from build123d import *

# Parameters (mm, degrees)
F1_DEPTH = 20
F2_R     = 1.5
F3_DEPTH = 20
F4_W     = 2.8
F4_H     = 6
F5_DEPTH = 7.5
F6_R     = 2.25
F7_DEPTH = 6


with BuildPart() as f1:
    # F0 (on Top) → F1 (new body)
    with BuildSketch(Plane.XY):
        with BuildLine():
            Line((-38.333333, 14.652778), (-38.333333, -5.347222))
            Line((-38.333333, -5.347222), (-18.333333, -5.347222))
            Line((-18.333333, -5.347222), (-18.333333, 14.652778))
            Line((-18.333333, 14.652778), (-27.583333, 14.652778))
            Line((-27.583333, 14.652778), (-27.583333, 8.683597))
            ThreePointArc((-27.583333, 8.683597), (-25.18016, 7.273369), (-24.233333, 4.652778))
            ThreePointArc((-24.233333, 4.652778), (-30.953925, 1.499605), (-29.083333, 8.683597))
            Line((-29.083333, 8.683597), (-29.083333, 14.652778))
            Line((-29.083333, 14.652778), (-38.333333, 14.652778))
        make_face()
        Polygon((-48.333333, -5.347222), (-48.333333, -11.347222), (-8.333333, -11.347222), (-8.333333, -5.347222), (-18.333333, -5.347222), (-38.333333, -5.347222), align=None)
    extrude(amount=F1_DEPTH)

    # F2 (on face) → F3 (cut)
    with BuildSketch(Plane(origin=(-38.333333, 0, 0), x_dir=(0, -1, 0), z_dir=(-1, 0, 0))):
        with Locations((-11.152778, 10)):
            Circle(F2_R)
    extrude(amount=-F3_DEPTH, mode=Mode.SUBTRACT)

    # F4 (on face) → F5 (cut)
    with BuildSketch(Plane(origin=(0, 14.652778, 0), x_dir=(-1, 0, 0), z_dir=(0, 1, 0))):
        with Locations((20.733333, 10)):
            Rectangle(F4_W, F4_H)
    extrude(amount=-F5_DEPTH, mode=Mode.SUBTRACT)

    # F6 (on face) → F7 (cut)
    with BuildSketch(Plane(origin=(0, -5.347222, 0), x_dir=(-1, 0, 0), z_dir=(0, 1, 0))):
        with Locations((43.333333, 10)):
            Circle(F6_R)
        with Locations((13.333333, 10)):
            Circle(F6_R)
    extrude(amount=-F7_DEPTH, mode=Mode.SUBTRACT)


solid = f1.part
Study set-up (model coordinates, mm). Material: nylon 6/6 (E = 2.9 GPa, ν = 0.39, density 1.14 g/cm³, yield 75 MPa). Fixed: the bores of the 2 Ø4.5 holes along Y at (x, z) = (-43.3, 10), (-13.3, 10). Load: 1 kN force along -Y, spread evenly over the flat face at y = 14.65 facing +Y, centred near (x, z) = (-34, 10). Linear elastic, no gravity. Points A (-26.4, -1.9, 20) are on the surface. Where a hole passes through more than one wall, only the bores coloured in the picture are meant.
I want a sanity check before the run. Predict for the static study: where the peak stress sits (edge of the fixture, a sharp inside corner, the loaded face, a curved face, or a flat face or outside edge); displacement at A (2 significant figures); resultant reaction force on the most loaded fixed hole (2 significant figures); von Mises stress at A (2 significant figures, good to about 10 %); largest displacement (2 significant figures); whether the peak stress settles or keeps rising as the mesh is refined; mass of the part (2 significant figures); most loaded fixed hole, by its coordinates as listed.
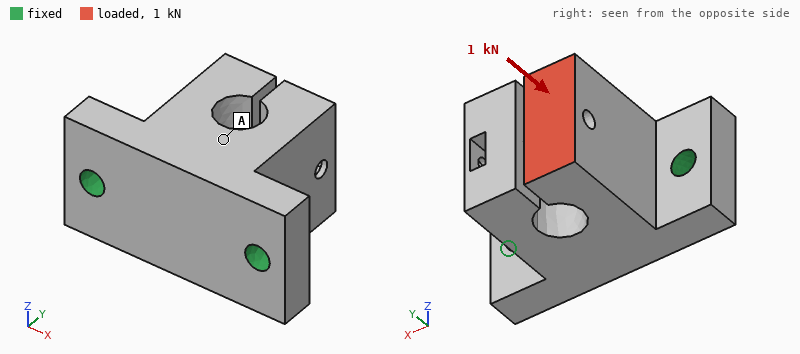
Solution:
edge of the fixture
0.065 mm
740 N
4.9 MPa
0.21 mm
keeps rising
13 g
(-43.3, 10)
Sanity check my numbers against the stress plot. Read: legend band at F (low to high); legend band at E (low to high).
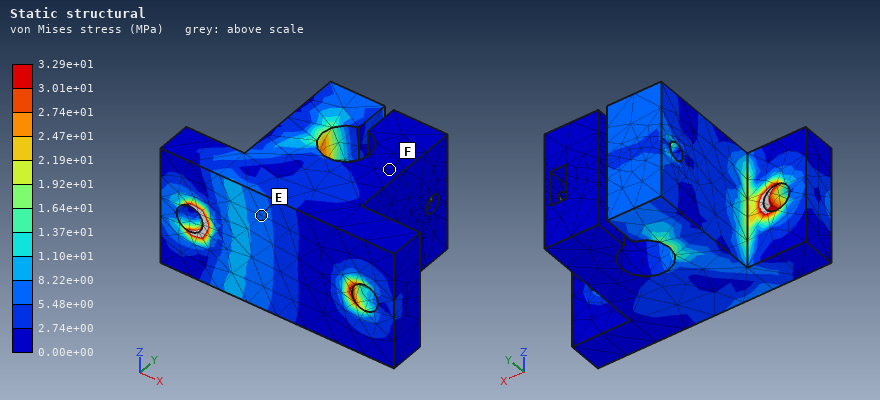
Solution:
0.00e+00 to 2.74e+00 MPa
5.48e+00 to 8.22e+00 MPa
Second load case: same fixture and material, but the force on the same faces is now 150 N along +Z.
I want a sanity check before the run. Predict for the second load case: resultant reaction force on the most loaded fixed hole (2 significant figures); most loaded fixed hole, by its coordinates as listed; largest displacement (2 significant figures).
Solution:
99 N
(-43.3, 10)
0.28 mm
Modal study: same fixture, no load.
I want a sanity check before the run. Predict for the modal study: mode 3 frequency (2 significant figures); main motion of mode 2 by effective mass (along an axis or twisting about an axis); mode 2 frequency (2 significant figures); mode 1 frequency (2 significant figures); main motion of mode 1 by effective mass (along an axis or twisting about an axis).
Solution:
4600 Hz
along X
4000 Hz
2300 Hz
along Z
